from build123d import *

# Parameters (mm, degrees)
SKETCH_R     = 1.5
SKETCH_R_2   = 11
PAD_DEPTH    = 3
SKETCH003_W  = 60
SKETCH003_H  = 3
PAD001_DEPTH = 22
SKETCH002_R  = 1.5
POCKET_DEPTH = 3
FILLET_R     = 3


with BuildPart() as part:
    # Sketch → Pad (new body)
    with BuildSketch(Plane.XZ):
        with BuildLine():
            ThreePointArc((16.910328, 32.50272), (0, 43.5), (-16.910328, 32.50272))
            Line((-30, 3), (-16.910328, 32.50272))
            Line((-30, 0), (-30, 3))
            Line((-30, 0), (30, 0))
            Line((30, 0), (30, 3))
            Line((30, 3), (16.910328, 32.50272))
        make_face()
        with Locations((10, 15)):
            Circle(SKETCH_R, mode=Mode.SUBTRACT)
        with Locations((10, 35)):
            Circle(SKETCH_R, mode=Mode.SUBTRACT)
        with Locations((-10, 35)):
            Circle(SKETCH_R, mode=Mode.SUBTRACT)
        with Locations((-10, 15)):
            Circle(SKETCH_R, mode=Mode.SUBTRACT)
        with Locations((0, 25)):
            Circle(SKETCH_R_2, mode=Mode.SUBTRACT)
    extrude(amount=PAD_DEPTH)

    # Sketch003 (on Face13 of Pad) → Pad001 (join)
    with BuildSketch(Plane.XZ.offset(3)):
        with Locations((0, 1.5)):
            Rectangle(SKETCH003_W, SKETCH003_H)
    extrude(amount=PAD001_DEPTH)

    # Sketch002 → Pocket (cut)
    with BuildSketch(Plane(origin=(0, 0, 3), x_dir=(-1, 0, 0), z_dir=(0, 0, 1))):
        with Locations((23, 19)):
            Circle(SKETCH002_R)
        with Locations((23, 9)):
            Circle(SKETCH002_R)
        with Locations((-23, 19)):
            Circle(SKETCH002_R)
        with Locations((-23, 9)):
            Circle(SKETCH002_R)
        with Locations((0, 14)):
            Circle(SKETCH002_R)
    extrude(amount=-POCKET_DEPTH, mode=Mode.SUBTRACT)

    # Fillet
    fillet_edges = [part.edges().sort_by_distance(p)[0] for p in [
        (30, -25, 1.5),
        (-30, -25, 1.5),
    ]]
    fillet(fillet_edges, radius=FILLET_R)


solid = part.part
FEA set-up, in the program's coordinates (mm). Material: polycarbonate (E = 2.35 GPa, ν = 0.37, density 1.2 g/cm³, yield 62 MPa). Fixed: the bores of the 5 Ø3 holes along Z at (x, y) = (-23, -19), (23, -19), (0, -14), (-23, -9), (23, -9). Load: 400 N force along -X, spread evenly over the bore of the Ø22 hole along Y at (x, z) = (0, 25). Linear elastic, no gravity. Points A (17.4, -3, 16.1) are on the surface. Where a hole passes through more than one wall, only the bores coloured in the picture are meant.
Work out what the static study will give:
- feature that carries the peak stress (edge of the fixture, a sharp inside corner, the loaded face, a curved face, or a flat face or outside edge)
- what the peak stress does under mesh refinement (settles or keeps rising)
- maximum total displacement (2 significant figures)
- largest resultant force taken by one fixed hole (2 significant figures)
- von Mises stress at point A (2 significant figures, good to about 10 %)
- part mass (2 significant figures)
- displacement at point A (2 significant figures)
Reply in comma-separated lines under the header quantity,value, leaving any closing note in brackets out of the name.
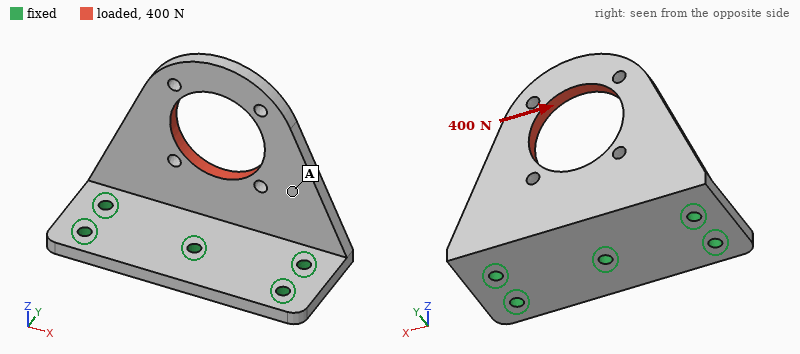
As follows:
quantity,value
feature that carries the peak stress,edge of the fixture
what the peak stress does under mesh refinement,keeps rising
maximum total displacement,0.92 mm
largest resultant force taken by one fixed hole,270 N
von Mises stress at point A,8.3 MPa
part mass,9.7 g
displacement at point A,0.47 mm
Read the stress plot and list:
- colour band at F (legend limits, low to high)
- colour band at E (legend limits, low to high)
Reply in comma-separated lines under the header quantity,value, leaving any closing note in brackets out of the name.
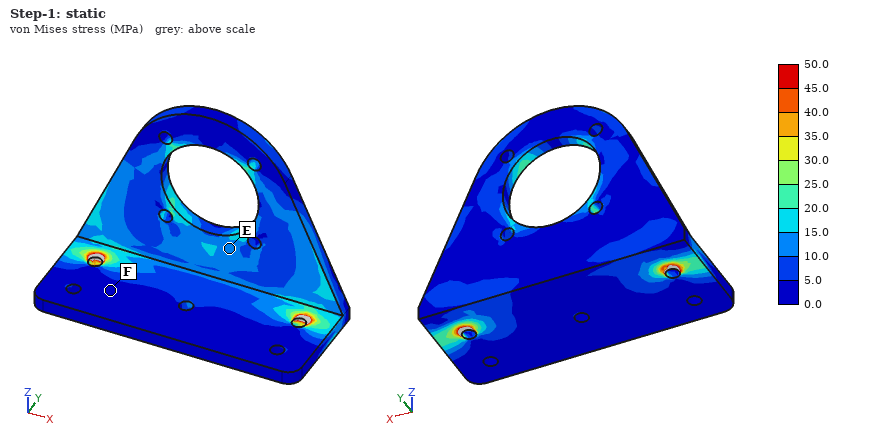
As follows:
quantity,value
colour band at F,0.0 to 5.0 MPa
colour band at E,10.0 to 15.0 MPa
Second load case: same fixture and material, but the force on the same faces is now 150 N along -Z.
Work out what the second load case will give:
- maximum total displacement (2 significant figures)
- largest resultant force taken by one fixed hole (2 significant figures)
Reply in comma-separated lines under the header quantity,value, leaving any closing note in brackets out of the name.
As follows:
quantity,value
maximum total displacement,0.73 mm
largest resultant force taken by one fixed hole,85 N
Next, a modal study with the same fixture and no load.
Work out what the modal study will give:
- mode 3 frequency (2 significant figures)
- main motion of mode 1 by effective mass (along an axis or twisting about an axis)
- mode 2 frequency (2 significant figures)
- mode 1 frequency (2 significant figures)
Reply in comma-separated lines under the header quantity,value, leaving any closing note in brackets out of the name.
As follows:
quantity,value
mode 3 frequency,1800 Hz
main motion of mode 1 by effective mass,along Y
mode 2 frequency,1100 Hz
mode 1 frequency,460 Hz
